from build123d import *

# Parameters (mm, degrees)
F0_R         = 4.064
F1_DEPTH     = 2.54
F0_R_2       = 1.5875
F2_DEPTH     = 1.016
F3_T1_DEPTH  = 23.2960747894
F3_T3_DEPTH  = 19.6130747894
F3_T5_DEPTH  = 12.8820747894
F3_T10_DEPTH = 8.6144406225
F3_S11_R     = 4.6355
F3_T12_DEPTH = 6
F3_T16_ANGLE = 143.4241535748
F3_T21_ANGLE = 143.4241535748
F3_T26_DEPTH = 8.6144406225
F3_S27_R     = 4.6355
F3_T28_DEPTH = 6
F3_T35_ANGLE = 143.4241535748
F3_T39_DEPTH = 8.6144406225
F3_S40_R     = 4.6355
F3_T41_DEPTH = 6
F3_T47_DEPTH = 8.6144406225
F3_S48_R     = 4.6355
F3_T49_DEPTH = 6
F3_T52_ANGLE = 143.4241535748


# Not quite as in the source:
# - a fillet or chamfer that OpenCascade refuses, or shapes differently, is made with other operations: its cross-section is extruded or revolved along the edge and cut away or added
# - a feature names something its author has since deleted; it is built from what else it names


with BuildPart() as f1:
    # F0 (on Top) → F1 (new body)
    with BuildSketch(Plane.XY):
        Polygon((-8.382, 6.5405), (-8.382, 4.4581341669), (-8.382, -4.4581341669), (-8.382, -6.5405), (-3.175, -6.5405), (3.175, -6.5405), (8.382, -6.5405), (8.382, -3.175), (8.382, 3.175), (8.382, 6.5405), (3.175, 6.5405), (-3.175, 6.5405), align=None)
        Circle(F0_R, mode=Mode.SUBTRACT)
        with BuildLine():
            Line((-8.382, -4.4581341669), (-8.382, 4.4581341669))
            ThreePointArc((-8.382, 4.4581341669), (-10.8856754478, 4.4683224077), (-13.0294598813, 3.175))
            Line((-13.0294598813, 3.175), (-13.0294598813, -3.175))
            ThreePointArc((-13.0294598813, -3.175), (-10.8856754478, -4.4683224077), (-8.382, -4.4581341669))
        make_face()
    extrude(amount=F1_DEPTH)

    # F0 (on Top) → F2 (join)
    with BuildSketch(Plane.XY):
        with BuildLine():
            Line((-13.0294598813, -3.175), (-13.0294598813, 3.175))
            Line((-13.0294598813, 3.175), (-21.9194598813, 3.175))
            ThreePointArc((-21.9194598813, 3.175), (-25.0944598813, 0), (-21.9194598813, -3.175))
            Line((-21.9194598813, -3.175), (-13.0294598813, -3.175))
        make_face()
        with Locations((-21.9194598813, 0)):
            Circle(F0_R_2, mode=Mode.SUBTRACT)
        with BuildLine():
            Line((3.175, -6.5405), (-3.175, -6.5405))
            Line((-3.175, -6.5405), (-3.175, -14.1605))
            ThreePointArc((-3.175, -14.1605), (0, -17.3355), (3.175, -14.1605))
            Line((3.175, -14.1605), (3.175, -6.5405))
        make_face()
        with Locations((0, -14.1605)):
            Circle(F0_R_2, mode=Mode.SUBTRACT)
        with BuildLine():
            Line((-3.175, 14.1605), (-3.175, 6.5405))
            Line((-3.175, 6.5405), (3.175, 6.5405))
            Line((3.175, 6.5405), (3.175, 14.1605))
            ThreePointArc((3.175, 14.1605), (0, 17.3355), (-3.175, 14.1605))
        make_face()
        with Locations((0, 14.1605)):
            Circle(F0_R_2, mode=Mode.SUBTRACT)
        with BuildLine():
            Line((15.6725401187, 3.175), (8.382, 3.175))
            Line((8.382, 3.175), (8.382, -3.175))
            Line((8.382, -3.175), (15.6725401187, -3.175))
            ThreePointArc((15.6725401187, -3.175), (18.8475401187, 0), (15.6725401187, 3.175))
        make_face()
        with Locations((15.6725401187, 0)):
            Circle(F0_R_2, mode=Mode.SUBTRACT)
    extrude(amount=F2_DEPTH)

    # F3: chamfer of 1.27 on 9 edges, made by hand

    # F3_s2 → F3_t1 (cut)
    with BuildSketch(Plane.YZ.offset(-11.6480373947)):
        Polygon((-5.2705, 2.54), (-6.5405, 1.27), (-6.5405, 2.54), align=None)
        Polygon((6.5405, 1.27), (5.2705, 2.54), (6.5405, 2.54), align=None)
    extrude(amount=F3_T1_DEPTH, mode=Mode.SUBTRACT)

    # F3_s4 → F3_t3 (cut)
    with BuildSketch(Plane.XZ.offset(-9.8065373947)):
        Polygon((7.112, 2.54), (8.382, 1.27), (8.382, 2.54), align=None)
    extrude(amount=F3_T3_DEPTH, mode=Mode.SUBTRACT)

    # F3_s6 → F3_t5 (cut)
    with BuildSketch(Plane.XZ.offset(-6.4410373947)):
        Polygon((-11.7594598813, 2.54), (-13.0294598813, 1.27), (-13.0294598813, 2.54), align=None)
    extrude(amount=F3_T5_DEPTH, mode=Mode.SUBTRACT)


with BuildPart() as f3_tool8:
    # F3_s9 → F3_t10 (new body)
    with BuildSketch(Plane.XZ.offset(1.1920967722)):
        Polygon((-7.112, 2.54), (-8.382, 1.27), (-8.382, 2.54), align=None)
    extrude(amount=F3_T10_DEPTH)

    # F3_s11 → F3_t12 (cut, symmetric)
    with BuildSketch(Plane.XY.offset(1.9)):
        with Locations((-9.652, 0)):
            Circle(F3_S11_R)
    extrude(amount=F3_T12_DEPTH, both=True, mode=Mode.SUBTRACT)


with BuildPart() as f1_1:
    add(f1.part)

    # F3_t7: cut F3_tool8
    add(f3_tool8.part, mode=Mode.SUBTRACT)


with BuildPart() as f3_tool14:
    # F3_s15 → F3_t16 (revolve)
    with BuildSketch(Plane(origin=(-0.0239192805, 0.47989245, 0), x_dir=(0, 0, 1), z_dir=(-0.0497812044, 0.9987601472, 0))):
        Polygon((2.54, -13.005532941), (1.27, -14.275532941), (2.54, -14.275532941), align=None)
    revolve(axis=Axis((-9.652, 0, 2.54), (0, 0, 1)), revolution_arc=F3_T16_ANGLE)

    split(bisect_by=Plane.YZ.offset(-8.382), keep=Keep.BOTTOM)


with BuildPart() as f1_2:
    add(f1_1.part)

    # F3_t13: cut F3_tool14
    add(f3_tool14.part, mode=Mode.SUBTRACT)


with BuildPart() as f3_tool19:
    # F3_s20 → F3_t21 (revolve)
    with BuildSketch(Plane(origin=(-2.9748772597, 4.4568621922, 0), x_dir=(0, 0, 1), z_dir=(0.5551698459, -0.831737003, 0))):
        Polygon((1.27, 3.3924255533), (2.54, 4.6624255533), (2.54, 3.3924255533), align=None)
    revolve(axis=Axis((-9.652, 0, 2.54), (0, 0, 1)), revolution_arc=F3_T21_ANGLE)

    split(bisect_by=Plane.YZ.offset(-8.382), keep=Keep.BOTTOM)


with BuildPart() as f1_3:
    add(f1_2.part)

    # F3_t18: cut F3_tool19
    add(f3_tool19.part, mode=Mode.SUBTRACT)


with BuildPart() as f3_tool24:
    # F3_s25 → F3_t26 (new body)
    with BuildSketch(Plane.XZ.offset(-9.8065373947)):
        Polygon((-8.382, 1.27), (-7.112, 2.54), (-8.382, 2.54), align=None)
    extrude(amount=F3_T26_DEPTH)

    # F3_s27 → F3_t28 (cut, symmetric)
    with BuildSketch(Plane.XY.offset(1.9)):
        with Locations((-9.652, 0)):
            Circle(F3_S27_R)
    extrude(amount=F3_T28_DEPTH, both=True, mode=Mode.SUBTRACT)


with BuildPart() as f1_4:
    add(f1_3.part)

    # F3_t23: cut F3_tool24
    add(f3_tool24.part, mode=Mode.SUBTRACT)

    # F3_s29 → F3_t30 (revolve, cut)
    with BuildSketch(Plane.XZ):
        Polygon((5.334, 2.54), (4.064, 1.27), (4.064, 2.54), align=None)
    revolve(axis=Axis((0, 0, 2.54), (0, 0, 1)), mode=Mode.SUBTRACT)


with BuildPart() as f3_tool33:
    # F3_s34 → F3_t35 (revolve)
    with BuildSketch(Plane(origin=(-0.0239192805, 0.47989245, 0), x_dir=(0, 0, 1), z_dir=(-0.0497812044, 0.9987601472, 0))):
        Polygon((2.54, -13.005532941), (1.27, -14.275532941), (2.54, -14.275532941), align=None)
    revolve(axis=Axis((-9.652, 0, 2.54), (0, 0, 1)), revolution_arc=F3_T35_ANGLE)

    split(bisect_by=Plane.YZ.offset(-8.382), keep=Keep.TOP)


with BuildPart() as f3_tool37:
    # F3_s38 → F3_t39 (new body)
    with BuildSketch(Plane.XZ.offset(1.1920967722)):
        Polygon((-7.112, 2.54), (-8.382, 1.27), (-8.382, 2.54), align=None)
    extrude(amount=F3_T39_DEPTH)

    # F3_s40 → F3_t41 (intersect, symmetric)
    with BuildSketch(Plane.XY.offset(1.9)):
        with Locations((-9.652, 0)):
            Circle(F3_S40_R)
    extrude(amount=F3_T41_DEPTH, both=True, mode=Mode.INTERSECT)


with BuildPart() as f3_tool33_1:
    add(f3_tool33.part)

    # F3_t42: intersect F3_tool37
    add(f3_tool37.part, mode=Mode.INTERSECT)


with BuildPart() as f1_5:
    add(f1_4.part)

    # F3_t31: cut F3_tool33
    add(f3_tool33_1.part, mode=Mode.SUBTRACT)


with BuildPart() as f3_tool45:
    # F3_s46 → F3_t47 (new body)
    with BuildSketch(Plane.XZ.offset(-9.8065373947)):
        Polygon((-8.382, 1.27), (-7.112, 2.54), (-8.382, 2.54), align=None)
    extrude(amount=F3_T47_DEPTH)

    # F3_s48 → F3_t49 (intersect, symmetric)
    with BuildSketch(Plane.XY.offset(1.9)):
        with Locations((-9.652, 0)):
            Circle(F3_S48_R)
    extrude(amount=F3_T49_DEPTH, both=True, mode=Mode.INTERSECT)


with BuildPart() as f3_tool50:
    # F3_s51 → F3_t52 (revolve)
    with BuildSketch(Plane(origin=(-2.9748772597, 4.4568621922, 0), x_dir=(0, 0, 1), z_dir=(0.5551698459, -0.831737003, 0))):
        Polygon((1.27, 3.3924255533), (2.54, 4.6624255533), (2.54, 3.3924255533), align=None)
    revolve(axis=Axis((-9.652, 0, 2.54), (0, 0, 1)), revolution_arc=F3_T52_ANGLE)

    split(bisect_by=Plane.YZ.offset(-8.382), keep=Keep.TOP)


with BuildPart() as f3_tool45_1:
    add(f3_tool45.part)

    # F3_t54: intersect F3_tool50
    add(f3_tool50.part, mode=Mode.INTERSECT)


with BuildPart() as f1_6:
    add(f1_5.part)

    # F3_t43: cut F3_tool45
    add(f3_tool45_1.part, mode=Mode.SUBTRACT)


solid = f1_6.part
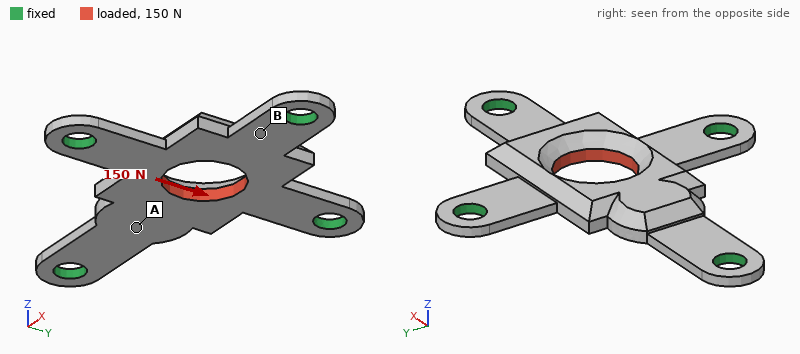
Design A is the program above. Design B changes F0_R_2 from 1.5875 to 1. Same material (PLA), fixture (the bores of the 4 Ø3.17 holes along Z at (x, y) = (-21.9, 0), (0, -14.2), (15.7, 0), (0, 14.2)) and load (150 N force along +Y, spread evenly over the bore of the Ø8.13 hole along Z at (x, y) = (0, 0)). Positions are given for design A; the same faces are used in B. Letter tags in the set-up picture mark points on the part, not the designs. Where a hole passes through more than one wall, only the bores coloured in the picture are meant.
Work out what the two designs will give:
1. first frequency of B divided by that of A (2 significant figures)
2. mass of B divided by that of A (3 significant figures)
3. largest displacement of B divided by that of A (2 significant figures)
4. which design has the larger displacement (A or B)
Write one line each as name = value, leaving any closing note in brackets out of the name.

first frequency of B divided by that of A = 0.88
mass of B divided by that of A = 1.03
largest displacement of B divided by that of A = 1.1
which design has the larger displacement = B
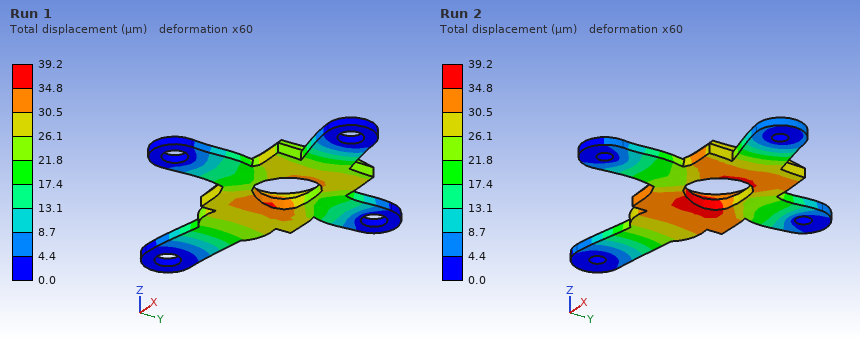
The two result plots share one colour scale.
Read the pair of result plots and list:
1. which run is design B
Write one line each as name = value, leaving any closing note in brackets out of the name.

which run is design B = Run 2
